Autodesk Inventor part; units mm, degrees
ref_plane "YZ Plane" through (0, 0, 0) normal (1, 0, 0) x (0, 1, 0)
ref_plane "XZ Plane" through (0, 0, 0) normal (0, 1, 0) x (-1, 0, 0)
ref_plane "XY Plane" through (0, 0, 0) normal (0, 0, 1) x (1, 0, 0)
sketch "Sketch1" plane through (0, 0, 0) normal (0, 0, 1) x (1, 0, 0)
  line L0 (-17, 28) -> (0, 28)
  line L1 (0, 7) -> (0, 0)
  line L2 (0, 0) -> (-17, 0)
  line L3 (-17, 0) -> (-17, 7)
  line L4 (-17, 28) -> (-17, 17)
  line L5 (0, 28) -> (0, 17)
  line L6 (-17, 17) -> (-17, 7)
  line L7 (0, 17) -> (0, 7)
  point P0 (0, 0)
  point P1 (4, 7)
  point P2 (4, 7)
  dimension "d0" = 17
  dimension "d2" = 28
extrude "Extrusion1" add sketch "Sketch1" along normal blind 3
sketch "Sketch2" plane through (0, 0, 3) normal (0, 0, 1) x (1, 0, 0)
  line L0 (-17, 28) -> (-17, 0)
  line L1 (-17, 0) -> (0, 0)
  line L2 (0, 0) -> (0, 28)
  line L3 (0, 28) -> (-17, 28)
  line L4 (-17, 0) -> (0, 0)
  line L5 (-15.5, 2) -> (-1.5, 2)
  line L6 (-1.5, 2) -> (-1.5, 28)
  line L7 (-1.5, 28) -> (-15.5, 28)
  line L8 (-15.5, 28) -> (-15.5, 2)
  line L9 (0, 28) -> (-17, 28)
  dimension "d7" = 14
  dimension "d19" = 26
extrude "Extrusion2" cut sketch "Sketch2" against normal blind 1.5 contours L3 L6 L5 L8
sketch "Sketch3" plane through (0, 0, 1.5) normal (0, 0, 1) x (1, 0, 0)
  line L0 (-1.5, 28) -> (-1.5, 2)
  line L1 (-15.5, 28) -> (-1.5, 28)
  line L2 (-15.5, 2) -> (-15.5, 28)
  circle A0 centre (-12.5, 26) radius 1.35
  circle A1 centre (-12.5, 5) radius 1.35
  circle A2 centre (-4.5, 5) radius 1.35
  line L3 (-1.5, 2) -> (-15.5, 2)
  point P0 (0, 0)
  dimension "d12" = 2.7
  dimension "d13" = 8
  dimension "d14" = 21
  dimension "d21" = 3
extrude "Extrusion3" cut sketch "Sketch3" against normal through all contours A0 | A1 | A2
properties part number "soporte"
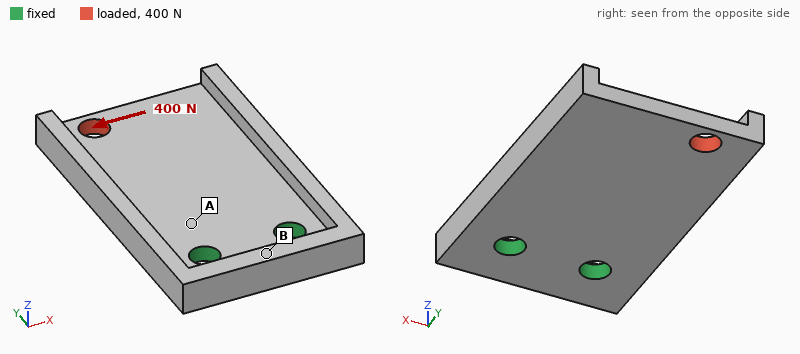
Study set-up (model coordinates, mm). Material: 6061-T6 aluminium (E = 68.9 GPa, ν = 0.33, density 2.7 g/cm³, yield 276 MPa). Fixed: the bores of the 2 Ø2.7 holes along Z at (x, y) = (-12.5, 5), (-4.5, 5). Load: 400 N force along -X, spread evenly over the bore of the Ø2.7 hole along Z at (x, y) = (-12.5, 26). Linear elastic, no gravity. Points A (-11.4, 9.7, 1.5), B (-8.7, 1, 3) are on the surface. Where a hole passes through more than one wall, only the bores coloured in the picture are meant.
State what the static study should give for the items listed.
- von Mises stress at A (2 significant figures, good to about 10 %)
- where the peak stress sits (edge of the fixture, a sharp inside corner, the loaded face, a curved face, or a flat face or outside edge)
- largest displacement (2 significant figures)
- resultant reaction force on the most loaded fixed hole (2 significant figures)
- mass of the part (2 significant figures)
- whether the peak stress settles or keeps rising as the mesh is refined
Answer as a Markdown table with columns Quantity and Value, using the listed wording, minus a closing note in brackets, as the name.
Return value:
| Quantity | Value |
|---|---|
| von Mises stress at A | 58 MPa |
| where the peak stress sits | edge of the fixture |
| largest displacement | 67 µm |
| resultant reaction force on the most loaded fixed hole | 850 N |
| mass of the part | 2.3 g |
| whether the peak stress settles or keeps rising as the mesh is refined | keeps rising |
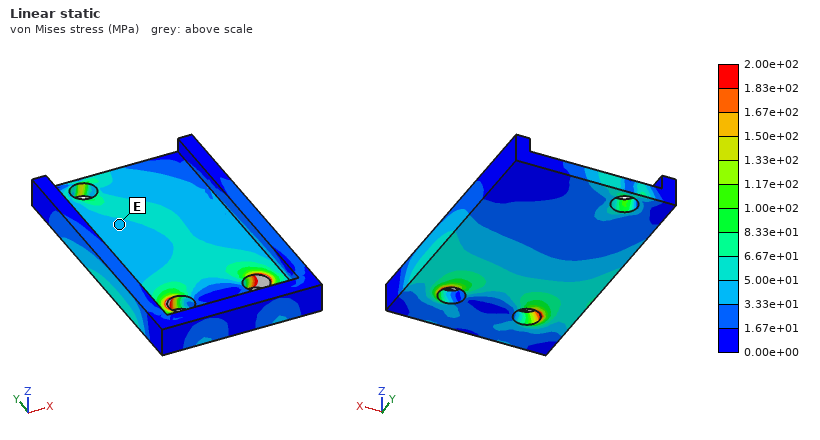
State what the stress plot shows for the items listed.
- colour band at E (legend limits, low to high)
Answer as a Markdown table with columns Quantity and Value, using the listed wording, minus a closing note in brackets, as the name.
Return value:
| Quantity | Value |
|---|---|
| colour band at E | 3.33e+01 to 5.00e+01 MPa |
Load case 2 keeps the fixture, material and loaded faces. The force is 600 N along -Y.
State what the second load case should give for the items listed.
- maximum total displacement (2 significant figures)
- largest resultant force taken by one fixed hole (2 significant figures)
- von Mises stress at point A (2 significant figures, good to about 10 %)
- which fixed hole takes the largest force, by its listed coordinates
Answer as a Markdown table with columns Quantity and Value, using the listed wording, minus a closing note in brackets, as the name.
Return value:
| Quantity | Value |
|---|---|
| maximum total displacement | 39 µm |
| largest resultant force taken by one fixed hole | 550 N |
| von Mises stress at point A | 35 MPa |
| which fixed hole takes the largest force, by its listed coordinates | (-12.5, 5) |
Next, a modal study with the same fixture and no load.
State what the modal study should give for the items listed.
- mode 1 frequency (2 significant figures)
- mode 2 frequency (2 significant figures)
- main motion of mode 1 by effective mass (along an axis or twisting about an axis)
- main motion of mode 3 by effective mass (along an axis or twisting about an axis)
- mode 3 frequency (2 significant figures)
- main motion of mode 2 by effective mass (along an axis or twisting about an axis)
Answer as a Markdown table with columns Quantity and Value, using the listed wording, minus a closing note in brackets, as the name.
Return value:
| Quantity | Value |
|---|---|
| mode 1 frequency | 3400 Hz |
| mode 2 frequency | 7000 Hz |
| main motion of mode 1 by effective mass | along Z |
| main motion of mode 3 by effective mass | along X |
| mode 3 frequency | 17 kHz |
| main motion of mode 2 by effective mass | twisting about Y |
